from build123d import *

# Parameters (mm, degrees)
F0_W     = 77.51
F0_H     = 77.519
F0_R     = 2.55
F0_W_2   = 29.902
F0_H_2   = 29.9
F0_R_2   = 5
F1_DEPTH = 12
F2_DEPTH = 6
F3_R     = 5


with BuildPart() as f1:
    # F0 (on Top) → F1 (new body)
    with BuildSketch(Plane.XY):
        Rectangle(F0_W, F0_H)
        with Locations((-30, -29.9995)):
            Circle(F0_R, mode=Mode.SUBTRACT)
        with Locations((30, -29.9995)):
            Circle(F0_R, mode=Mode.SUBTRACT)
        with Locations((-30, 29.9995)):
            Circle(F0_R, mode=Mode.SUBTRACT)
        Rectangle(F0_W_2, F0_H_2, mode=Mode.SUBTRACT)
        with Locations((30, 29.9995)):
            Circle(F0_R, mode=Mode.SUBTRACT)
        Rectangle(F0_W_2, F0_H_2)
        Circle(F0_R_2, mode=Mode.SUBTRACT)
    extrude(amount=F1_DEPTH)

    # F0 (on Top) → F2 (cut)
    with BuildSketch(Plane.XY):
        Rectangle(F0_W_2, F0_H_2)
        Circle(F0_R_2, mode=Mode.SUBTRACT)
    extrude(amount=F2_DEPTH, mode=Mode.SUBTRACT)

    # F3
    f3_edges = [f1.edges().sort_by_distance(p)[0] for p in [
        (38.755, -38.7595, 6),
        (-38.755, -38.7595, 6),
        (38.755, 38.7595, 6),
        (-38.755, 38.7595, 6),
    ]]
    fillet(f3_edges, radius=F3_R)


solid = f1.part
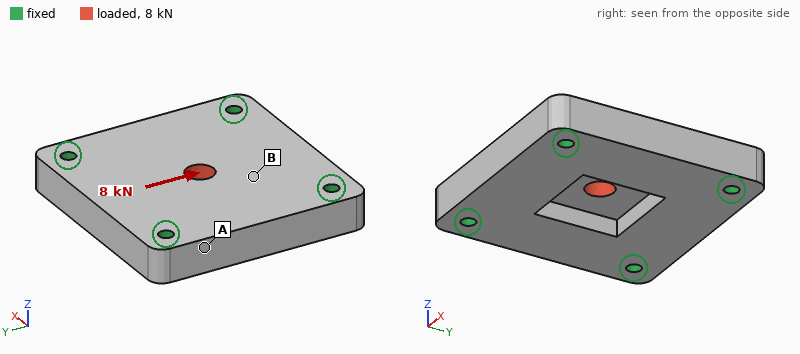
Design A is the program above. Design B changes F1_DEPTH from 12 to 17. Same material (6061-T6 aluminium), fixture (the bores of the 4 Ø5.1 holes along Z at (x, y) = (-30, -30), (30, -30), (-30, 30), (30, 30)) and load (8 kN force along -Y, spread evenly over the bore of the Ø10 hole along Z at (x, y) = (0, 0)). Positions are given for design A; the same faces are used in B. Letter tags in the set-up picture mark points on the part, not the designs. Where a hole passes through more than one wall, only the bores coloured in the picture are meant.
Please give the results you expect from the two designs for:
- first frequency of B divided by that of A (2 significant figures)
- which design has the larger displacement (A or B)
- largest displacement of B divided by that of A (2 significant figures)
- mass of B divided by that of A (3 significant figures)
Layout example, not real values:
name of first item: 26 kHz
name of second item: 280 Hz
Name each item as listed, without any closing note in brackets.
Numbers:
first frequency of B divided by that of A: 1.2
which design has the larger displacement: A
largest displacement of B divided by that of A: 0.62
mass of B divided by that of A: 1.45
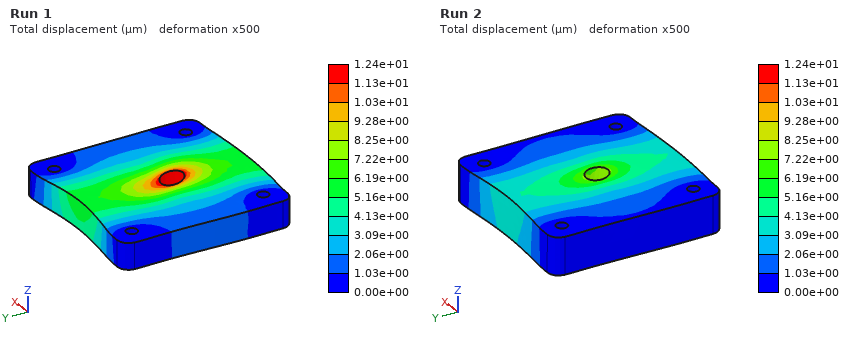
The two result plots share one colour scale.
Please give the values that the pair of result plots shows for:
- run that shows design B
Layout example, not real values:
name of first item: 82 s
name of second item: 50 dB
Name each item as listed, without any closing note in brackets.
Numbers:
run that shows design B: Run 2
